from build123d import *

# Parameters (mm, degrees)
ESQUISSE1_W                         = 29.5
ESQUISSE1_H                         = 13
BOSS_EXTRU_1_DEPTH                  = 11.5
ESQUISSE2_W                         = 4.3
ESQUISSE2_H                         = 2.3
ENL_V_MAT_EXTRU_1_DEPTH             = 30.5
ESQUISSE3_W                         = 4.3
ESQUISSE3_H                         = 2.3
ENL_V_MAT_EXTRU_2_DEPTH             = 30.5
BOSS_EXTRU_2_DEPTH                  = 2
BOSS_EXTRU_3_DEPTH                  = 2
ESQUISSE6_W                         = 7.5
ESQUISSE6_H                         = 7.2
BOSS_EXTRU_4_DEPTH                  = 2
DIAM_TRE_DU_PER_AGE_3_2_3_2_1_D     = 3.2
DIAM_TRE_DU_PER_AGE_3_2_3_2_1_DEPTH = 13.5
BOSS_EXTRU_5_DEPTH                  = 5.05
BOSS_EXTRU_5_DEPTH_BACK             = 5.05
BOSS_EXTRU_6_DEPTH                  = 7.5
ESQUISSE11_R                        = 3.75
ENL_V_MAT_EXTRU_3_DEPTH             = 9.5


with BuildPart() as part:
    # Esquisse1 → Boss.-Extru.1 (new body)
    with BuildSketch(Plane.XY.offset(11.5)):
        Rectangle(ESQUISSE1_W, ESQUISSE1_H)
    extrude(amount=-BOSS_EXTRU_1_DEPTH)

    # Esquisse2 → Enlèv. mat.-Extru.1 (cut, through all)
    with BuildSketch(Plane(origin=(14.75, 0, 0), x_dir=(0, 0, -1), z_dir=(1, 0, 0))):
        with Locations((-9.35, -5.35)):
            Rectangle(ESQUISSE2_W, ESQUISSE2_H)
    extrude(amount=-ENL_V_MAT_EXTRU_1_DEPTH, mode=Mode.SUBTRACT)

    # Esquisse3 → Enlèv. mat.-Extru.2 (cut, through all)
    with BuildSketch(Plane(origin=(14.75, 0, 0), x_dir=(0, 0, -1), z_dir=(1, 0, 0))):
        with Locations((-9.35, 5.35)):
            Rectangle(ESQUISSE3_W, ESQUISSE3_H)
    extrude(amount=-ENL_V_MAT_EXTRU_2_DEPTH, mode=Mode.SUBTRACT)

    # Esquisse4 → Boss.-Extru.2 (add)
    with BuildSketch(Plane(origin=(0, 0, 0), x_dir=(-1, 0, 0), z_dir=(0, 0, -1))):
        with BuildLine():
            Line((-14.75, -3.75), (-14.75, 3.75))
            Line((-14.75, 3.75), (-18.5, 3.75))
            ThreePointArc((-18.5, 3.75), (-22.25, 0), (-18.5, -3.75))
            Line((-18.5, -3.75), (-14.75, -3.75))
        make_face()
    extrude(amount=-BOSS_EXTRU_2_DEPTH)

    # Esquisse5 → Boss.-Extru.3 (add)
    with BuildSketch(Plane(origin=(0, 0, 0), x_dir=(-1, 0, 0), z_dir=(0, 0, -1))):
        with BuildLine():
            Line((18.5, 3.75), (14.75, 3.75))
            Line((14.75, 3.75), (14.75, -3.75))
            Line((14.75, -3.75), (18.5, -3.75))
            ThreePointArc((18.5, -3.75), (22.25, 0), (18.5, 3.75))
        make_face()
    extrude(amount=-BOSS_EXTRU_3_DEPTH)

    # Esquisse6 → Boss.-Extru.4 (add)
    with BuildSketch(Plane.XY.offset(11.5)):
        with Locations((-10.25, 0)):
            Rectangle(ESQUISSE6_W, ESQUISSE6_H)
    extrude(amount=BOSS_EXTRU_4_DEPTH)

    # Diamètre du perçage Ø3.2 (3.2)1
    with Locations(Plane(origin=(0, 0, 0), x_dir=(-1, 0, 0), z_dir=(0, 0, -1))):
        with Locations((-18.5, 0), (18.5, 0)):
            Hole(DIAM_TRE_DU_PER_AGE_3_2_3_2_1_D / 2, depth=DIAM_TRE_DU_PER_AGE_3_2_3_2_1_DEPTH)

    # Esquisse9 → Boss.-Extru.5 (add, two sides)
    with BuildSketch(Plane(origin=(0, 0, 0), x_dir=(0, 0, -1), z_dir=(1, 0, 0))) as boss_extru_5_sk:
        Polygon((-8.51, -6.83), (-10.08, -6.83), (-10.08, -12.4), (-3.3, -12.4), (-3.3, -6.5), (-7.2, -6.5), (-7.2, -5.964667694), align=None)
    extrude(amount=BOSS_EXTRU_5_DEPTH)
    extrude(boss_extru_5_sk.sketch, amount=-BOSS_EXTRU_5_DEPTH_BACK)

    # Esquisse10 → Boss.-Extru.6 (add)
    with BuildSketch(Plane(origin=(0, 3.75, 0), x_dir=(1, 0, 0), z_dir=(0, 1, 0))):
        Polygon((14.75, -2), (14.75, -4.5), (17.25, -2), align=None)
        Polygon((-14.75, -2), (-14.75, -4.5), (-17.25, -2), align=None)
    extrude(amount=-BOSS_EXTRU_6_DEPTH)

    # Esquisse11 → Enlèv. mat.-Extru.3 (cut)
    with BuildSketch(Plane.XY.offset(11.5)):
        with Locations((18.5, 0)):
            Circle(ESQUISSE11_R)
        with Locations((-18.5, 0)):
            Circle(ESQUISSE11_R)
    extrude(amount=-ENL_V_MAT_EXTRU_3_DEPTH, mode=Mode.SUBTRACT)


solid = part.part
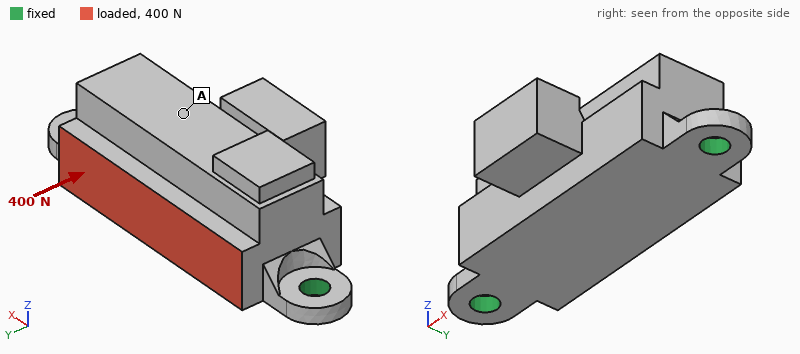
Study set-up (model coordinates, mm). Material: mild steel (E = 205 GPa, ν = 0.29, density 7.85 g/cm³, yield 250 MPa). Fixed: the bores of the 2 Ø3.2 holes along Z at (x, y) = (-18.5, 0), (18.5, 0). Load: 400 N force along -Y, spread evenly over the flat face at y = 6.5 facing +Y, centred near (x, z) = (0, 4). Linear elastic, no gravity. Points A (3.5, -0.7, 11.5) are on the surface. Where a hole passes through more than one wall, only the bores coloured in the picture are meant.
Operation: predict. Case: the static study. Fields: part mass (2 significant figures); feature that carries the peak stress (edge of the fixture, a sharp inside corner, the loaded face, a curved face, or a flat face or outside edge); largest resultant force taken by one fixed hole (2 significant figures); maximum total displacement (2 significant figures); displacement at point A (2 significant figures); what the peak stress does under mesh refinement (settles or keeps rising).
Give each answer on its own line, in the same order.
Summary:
36 g
edge of the fixture
200 N
10.0 µm
7.7 µm
keeps rising
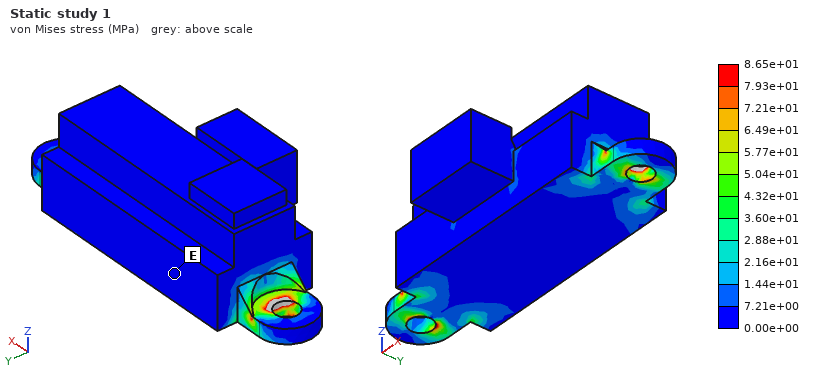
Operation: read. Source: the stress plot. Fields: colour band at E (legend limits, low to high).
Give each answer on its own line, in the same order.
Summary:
0.00e+00 to 7.21e+00 MPa
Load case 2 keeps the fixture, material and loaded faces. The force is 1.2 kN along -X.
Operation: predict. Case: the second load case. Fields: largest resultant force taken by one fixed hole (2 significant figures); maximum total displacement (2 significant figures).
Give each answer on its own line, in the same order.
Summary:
650 N
2.5 µm
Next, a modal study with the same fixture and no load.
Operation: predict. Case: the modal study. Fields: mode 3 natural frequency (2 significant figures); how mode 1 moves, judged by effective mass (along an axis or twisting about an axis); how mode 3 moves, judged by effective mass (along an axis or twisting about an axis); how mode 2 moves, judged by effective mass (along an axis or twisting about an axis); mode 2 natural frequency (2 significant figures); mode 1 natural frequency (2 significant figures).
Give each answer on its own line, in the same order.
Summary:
19 kHz
along Y
along Y
along Z
13 kHz
4900 Hz
